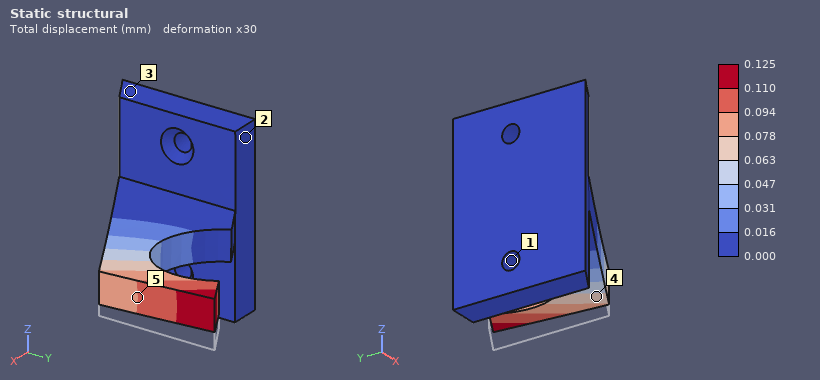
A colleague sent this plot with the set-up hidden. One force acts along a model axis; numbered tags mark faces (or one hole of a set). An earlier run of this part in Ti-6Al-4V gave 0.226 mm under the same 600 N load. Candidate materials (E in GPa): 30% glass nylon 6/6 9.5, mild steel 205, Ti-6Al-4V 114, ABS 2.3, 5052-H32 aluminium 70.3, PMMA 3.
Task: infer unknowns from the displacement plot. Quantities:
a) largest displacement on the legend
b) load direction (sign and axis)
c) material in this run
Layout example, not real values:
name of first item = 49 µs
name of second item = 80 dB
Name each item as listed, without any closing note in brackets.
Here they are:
largest displacement on the legend = 0.125 mm
load direction = +Z
material in this run = mild steel
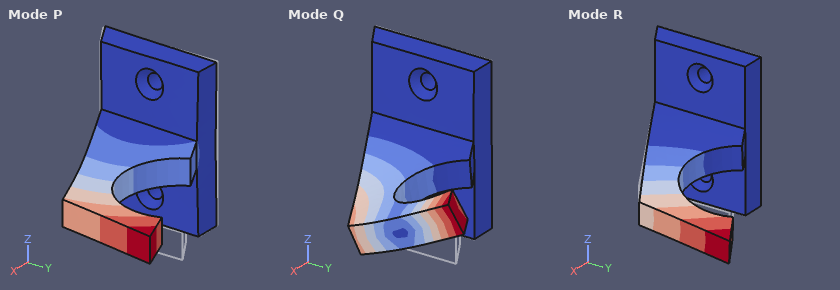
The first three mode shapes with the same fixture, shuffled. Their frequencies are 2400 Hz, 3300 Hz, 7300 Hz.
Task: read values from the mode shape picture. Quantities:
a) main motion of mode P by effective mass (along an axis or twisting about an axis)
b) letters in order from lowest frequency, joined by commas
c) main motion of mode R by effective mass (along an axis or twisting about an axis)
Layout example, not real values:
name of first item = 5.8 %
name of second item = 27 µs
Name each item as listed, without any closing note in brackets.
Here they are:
main motion of mode P by effective mass = along Y
letters in order from lowest frequency, joined by commas = R, P, Q
main motion of mode R by effective mass = along Z
